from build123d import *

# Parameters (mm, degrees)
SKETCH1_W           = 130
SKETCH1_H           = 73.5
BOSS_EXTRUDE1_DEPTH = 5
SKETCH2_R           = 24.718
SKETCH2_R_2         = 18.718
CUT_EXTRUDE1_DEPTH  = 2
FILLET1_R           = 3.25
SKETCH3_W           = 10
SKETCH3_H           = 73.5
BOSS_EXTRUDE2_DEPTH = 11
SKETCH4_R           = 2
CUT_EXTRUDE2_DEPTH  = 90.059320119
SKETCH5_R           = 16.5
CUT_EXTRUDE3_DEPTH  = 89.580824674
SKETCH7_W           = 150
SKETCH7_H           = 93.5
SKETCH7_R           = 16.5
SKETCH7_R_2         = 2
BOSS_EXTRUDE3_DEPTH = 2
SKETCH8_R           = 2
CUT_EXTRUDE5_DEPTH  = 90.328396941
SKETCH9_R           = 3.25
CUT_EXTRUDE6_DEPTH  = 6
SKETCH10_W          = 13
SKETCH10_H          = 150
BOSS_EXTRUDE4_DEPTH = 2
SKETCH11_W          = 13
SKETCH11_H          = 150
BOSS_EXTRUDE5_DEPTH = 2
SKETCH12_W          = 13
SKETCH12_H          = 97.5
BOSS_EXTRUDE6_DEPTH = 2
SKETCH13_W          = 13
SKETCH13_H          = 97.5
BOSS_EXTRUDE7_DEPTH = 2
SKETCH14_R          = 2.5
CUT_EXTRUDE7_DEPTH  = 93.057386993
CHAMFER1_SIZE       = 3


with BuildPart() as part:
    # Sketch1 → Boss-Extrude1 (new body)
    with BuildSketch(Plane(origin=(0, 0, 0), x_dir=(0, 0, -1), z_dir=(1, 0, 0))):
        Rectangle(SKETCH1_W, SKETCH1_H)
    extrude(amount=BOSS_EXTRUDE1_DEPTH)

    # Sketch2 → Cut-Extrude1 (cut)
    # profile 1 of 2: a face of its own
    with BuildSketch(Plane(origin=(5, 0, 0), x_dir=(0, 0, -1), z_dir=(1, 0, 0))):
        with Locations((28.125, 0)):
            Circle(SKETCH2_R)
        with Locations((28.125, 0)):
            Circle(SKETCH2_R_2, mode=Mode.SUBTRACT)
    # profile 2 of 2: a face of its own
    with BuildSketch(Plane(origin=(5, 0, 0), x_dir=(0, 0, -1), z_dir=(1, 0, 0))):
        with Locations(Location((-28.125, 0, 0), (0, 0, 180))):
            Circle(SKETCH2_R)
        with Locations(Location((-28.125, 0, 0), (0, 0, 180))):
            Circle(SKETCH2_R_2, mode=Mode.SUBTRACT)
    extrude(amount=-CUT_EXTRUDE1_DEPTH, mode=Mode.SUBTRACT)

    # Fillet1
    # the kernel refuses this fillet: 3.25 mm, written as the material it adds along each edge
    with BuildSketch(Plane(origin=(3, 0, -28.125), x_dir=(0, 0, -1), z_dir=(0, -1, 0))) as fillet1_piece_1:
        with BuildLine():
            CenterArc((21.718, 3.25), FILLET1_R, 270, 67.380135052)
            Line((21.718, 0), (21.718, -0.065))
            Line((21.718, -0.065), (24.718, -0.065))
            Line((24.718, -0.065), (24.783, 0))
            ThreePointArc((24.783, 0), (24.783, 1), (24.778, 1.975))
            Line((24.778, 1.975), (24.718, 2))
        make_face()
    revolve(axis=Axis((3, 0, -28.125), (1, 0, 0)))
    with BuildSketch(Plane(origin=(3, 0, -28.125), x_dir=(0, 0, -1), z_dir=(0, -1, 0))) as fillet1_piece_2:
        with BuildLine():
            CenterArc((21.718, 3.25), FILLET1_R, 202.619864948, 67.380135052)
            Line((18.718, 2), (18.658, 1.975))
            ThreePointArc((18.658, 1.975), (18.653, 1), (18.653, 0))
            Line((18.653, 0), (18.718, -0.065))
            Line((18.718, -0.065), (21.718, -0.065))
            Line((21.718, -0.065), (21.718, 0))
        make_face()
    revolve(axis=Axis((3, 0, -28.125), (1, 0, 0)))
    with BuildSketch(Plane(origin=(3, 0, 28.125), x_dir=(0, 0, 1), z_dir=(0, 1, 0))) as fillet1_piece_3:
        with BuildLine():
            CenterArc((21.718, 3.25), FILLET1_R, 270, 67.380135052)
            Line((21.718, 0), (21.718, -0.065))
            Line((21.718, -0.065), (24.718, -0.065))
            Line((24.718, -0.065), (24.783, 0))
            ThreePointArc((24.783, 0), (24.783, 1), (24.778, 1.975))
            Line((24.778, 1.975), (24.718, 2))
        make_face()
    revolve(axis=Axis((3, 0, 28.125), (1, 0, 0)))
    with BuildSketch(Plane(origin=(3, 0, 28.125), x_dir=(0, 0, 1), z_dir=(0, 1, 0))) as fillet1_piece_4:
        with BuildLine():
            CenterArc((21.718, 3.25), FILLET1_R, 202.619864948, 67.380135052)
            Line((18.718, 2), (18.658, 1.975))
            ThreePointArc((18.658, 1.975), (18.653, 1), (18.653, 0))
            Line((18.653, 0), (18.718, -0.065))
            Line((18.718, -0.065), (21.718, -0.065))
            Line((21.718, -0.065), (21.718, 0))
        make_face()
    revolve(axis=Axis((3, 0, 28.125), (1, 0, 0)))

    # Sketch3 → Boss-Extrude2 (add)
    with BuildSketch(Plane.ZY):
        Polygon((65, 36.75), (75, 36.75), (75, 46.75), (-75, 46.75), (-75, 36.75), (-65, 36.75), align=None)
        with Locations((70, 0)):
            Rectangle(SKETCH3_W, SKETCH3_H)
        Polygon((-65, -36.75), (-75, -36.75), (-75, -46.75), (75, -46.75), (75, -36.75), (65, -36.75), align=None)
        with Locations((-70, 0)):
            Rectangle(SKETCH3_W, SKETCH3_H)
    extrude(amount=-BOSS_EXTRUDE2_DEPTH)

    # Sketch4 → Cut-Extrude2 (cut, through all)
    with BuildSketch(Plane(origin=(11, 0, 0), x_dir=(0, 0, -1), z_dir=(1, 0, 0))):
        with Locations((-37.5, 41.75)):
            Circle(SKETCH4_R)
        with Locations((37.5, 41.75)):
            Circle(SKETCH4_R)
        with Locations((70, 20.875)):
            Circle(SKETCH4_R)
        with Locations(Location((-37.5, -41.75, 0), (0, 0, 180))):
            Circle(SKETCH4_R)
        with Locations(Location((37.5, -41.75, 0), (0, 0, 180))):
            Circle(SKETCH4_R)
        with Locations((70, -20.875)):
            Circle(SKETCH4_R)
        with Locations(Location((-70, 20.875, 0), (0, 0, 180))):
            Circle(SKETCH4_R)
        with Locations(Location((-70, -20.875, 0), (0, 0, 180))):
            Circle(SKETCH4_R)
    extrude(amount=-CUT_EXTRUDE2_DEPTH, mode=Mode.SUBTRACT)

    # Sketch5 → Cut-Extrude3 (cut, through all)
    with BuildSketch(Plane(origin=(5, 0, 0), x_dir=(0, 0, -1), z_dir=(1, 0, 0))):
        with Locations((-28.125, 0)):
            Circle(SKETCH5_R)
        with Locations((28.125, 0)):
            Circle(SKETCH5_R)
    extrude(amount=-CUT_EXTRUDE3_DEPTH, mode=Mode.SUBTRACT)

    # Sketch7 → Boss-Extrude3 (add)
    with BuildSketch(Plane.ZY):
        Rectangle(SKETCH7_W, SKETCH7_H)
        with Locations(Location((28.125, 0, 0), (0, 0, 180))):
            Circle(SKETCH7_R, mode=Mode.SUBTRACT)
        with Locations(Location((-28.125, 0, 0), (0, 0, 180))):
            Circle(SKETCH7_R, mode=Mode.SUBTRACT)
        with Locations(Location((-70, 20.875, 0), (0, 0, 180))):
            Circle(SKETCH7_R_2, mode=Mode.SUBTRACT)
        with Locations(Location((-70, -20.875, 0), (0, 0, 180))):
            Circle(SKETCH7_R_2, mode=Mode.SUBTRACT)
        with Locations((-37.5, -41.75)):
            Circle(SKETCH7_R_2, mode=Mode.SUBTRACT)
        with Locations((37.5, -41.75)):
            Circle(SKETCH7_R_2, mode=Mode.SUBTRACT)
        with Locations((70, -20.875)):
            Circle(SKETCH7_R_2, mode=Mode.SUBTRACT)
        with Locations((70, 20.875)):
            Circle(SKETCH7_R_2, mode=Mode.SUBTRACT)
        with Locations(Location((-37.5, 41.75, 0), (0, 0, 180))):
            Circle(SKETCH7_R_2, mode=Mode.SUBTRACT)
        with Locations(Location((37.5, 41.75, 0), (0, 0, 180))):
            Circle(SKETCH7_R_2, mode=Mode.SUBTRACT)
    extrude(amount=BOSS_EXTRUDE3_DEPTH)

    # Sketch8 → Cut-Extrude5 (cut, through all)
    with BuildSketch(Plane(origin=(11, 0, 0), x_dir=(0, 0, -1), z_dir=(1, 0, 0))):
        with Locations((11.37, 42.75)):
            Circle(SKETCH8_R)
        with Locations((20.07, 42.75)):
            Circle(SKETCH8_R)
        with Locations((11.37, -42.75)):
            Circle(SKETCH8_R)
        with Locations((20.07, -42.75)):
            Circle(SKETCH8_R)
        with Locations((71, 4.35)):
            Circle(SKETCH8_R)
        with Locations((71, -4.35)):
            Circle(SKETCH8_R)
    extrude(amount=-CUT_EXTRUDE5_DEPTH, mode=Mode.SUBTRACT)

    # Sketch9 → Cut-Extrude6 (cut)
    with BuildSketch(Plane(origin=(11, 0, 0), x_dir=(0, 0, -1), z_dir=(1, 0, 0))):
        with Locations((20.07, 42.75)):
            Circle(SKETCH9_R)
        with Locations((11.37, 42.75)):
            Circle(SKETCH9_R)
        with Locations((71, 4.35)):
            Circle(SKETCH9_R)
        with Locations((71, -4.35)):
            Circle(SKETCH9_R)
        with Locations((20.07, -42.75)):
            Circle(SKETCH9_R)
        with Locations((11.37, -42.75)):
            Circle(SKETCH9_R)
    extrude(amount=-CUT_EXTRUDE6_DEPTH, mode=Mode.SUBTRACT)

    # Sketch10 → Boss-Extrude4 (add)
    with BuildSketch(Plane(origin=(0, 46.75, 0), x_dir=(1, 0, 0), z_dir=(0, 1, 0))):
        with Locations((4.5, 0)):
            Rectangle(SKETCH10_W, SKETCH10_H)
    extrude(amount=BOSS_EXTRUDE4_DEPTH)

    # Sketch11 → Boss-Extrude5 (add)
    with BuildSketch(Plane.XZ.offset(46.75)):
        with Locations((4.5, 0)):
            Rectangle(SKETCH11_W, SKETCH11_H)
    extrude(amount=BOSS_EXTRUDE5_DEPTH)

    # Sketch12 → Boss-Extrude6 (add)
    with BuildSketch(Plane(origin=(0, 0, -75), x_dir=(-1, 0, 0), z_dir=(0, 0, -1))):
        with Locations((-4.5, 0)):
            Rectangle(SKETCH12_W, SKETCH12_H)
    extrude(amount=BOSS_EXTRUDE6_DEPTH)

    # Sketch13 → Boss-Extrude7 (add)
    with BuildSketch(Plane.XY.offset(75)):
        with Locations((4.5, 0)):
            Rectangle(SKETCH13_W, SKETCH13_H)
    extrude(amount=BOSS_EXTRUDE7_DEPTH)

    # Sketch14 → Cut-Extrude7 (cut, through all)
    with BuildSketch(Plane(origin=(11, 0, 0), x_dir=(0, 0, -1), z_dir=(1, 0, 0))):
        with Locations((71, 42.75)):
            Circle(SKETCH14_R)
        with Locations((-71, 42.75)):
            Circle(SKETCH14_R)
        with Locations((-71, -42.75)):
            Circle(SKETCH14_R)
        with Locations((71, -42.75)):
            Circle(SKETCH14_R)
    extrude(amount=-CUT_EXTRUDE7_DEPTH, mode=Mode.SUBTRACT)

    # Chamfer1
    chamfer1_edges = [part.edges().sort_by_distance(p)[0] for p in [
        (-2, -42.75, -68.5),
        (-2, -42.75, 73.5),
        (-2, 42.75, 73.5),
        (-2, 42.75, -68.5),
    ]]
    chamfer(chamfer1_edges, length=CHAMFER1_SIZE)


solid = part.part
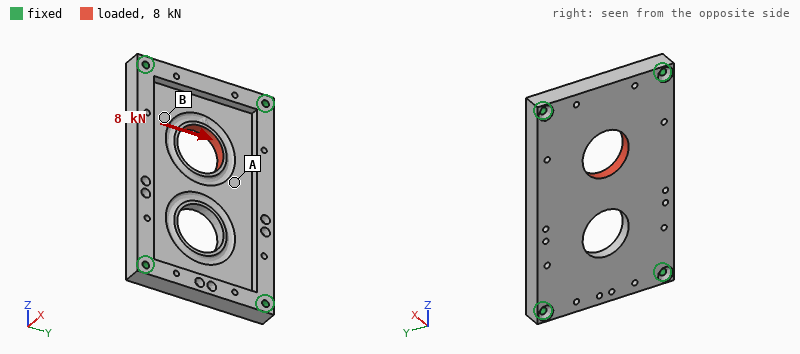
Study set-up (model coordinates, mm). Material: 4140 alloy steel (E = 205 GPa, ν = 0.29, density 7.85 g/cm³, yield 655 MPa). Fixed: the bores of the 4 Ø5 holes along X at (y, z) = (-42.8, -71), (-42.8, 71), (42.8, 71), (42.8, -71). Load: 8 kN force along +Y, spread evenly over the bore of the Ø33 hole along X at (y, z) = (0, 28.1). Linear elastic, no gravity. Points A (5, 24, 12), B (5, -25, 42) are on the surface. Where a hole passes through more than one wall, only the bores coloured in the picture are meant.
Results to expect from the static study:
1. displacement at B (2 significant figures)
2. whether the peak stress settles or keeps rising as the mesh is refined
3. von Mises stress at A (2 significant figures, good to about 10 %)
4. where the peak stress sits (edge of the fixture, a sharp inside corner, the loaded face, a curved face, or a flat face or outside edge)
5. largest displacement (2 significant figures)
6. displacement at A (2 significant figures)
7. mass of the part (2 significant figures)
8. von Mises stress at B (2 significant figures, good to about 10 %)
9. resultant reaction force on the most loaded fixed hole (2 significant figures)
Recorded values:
5.5 µm
keeps rising
7.3 MPa
edge of the fixture
9.8 µm
9.0 µm
930 g
15 MPa
3.3 kN
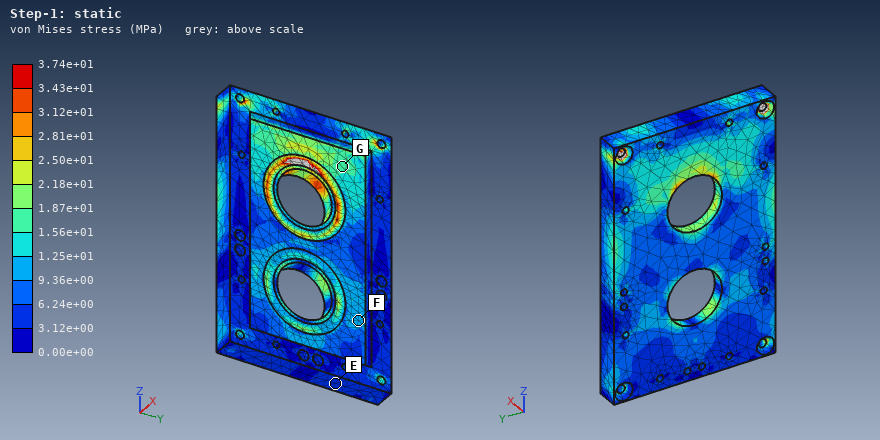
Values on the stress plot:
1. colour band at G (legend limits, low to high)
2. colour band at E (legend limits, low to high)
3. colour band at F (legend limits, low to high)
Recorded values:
1.56e+01 to 1.87e+01 MPa
3.12e+00 to 6.24e+00 MPa
9.36e+00 to 1.25e+01 MPa
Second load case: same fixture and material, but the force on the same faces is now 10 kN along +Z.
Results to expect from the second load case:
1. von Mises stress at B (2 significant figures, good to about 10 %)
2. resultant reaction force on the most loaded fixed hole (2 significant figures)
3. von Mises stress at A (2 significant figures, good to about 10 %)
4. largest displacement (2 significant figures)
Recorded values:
13 MPa
3.3 kN
14 MPa
8.1 µm
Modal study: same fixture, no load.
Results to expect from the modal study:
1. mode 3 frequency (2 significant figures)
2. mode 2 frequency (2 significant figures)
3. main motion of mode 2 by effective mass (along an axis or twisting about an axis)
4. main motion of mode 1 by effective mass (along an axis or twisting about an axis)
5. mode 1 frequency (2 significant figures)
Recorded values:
5000 Hz
3100 Hz
twisting about Z
along X
2300 Hz
